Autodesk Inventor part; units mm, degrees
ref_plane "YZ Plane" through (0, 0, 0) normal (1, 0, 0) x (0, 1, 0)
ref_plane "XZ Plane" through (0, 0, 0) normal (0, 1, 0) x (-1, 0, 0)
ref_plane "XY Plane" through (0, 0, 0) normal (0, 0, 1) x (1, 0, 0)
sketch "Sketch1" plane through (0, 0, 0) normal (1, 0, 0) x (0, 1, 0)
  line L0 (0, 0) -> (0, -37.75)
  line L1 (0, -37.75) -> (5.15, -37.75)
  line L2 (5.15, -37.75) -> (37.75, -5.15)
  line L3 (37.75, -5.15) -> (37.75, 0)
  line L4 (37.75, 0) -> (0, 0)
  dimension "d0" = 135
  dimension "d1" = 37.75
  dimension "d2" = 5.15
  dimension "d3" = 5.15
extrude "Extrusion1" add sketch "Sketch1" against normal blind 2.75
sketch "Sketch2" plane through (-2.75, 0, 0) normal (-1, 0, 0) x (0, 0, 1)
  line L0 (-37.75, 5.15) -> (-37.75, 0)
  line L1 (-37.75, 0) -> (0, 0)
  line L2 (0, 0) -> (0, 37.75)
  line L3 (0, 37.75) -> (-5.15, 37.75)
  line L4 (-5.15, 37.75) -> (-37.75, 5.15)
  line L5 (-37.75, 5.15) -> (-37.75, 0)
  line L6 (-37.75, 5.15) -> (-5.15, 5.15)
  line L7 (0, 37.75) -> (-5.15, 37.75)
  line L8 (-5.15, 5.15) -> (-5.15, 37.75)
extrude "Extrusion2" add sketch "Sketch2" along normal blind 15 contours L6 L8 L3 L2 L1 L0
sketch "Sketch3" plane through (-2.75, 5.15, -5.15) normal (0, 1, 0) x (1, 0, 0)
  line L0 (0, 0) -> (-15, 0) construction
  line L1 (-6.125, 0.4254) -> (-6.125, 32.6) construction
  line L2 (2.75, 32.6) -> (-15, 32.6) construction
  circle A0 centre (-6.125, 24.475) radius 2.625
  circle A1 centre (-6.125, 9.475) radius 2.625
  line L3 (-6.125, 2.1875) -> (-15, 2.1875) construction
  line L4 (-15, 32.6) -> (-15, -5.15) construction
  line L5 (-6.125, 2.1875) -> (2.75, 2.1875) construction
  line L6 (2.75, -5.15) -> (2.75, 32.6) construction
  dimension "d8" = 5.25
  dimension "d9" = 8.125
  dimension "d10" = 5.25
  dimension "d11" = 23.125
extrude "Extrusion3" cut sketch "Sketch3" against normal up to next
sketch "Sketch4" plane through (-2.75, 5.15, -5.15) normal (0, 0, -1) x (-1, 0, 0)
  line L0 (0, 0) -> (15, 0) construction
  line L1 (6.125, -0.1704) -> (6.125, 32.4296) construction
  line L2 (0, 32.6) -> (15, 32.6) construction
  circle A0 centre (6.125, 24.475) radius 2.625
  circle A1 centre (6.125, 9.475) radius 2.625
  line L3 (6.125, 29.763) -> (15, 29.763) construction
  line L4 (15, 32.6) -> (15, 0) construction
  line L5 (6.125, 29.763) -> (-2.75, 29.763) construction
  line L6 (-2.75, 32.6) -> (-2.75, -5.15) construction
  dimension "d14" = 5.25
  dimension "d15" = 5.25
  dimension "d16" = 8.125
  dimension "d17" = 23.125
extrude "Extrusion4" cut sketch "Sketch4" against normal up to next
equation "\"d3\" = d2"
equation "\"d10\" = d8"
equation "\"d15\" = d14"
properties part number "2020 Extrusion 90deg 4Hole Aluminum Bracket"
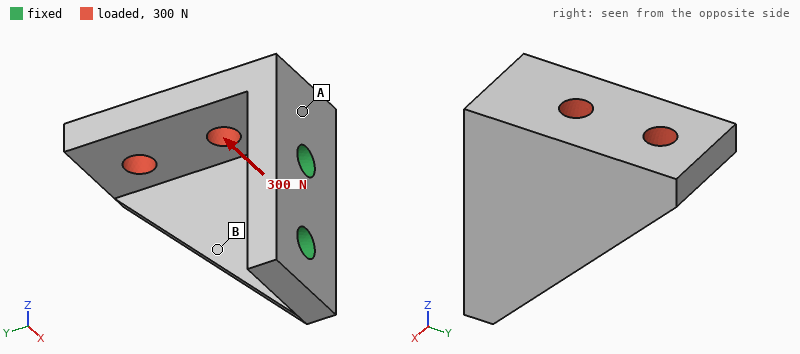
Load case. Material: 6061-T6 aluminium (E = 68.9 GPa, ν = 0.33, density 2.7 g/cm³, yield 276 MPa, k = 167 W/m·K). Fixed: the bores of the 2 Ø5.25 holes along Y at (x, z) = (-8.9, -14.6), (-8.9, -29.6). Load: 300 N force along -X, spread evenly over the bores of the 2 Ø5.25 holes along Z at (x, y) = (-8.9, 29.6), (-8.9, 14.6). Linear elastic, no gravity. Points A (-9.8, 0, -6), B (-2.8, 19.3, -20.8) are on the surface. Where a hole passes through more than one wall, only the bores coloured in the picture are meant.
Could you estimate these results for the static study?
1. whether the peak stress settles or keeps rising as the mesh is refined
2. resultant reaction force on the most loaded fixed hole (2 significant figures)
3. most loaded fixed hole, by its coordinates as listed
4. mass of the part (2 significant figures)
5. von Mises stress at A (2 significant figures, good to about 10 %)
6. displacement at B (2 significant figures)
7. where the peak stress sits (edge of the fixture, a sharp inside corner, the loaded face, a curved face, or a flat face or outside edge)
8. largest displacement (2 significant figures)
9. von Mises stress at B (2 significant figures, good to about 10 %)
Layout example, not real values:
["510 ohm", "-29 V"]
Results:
["keeps rising", "420 N", "(-8.9, -14.6)", "20 g", "25 MPa", "26 µm", "edge of the fixture", "83 µm", "10 MPa"]
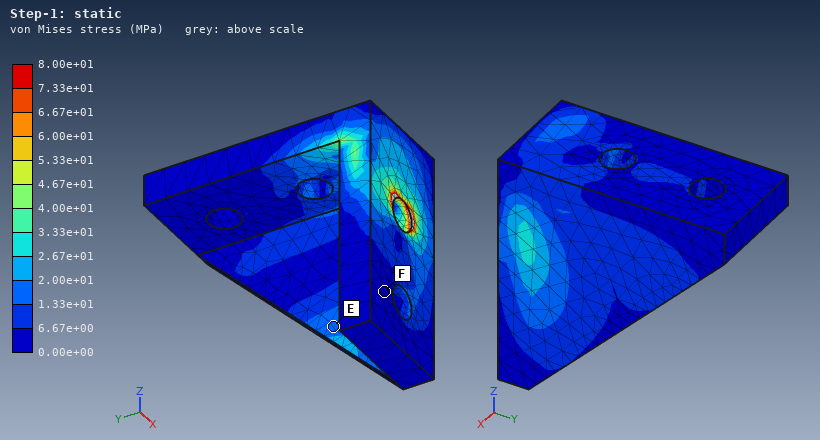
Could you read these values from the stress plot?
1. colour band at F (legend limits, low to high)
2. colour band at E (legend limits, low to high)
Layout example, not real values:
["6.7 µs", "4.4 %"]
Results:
["0.00e+00 to 6.67e+00 MPa", "1.33e+01 to 2.00e+01 MPa"]
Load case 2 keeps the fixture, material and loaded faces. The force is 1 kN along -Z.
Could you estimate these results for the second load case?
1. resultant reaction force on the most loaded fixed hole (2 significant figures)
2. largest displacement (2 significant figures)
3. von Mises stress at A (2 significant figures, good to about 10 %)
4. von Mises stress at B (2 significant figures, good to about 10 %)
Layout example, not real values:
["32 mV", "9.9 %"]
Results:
["980 N", "0.19 mm", "36 MPa", "50 MPa"]
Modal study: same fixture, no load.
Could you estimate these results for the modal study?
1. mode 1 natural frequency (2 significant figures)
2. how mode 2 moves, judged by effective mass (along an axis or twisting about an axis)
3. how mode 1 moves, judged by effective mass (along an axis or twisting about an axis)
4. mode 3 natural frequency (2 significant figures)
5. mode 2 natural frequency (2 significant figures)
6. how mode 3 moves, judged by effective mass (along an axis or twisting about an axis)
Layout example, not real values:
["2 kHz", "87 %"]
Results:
["3800 Hz", "along Z", "along X", "11 kHz", "5700 Hz", "along Y"]
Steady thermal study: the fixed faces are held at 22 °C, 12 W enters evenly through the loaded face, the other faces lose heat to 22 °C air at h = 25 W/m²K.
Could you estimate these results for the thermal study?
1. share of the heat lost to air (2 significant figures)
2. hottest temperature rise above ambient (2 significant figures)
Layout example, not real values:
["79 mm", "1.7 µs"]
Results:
["5.8 %", "16 K"]
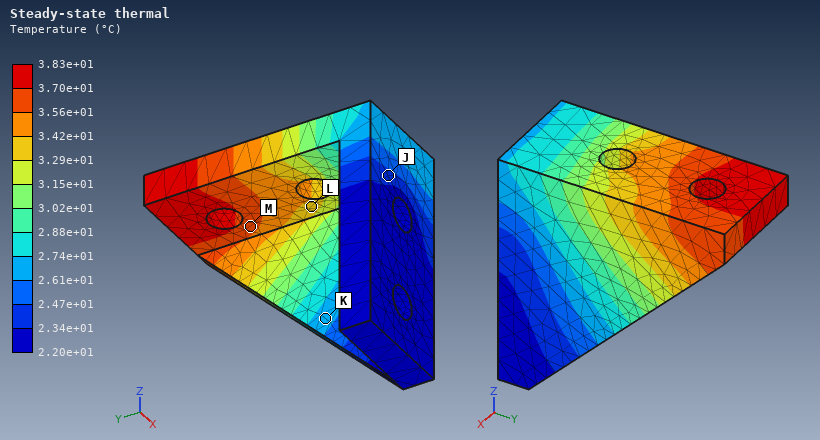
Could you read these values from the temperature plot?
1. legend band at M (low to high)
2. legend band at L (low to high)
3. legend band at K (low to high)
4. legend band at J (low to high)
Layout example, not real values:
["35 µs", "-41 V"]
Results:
["3.56e+01 to 3.70e+01 °C", "3.29e+01 to 3.42e+01 °C", "2.61e+01 to 2.74e+01 °C", "2.34e+01 to 2.47e+01 °C"]
